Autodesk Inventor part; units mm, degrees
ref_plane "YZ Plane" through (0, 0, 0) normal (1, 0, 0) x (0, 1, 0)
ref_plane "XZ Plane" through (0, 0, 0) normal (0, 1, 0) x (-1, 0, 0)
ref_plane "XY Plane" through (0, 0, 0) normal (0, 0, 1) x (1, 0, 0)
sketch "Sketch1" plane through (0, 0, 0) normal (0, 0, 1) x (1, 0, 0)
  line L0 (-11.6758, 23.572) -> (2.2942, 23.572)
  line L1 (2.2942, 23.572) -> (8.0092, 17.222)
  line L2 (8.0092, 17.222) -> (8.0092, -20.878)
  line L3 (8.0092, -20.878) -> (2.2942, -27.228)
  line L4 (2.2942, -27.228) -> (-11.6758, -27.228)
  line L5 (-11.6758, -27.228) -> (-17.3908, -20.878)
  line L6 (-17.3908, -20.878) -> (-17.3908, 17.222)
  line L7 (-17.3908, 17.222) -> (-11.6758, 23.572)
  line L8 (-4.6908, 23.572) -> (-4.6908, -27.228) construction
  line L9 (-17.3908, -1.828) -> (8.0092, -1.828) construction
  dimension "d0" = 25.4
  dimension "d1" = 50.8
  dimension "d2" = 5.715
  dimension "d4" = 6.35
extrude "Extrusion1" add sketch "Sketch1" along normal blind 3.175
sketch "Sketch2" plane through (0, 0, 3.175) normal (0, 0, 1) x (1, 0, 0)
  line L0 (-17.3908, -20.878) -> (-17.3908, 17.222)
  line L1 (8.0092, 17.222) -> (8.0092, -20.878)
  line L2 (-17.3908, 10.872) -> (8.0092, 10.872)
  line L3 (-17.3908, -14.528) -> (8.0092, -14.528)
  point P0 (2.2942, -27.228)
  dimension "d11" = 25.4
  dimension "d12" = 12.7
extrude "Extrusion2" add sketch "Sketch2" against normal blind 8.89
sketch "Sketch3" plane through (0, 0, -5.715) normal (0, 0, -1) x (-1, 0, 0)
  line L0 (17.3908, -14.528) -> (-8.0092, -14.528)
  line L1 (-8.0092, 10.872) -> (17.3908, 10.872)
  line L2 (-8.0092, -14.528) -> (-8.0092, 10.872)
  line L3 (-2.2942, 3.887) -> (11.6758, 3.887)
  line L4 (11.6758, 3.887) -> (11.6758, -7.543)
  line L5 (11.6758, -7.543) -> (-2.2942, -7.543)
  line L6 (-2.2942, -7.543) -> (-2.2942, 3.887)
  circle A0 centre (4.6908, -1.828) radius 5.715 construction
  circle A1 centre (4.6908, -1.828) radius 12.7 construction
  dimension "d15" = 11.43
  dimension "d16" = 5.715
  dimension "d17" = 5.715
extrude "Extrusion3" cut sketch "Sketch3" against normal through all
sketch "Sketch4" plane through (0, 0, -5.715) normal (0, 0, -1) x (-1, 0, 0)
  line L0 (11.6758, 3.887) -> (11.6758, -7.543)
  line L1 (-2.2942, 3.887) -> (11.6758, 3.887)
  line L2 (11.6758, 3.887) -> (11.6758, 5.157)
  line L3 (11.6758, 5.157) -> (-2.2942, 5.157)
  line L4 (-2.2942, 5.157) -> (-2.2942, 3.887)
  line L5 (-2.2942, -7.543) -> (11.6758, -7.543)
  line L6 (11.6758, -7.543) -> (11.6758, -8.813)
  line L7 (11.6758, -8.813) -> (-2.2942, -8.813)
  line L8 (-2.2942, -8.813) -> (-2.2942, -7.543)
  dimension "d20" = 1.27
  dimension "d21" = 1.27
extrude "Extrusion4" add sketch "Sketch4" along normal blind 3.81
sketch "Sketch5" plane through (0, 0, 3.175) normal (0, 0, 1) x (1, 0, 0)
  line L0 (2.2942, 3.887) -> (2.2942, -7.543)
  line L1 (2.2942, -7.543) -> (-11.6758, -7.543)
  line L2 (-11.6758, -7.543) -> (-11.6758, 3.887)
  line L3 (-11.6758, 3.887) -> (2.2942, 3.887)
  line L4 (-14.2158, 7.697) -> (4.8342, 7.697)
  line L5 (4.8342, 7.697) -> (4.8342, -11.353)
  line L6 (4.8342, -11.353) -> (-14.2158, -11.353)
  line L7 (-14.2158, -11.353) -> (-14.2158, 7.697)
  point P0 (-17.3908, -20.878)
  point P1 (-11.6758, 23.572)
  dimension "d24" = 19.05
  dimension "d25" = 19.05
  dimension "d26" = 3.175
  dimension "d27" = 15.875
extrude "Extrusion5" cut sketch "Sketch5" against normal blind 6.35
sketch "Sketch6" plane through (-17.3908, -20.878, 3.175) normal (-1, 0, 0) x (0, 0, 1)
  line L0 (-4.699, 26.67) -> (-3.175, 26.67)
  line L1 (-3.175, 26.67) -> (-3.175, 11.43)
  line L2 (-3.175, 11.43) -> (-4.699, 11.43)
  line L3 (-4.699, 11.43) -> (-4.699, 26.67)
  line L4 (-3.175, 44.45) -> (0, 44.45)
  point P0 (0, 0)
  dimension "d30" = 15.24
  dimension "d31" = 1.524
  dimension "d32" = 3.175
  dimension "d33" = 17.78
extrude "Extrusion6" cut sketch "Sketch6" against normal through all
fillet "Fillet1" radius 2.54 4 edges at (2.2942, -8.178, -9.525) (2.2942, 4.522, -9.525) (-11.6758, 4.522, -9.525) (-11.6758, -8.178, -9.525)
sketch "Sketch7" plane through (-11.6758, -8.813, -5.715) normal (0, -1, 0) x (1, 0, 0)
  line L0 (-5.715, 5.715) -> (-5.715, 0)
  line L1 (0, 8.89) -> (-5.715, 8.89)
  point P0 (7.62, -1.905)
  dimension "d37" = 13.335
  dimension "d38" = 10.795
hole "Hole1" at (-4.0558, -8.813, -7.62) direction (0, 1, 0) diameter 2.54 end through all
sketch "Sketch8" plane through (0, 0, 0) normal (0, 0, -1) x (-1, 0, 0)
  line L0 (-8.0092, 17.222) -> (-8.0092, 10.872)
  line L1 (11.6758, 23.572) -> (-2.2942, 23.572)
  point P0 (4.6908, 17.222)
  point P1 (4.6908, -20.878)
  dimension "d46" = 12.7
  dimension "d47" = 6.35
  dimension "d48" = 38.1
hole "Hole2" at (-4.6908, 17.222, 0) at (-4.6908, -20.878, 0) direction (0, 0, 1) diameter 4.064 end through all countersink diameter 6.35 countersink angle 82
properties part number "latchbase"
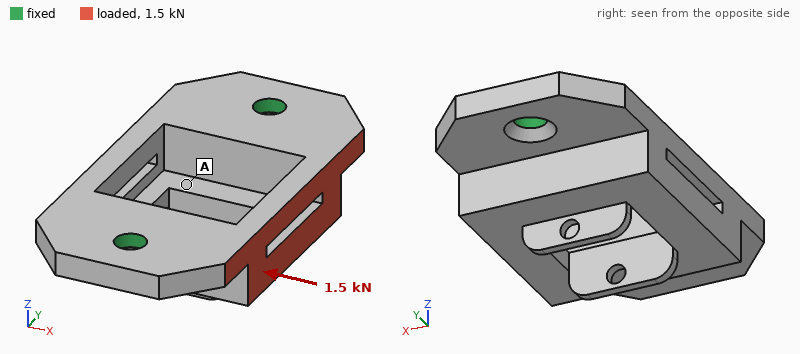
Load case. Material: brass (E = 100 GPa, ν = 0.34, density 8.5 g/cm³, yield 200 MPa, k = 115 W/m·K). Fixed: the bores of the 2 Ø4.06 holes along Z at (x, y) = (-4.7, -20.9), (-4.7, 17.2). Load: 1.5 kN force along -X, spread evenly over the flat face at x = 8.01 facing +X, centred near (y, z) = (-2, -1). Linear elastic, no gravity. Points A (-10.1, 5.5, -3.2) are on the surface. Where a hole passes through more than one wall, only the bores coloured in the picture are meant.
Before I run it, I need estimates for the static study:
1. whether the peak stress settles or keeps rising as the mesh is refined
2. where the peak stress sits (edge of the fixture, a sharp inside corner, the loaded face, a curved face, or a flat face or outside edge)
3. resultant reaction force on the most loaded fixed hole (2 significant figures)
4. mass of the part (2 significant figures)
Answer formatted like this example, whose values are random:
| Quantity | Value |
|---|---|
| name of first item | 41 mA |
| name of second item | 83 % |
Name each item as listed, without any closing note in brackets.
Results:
| Quantity | Value |
|---|---|
| whether the peak stress settles or keeps rising as the mesh is refined | keeps rising |
| where the peak stress sits | edge of the fixture |
| resultant reaction force on the most loaded fixed hole | 760 N |
| mass of the part | 40 g |
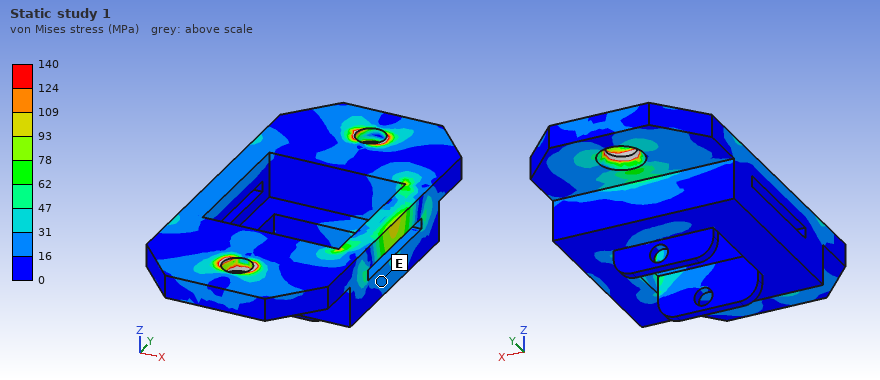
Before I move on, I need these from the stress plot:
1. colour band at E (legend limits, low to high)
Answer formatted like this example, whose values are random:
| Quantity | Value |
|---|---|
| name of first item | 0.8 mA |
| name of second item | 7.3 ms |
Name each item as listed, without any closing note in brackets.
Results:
| Quantity | Value |
|---|---|
| colour band at E | 16 to 31 MPa |
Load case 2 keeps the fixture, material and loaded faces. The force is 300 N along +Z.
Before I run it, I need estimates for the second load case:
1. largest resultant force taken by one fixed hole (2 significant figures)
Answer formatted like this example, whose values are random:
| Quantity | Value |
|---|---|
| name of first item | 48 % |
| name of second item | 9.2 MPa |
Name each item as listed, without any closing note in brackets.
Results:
| Quantity | Value |
|---|---|
| largest resultant force taken by one fixed hole | 210 N |
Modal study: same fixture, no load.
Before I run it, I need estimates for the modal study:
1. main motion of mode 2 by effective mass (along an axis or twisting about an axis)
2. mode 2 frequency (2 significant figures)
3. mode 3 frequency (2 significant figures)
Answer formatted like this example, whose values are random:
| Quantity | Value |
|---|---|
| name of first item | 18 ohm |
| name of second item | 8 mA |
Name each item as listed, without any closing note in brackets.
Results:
| Quantity | Value |
|---|---|
| main motion of mode 2 by effective mass | along Z |
| mode 2 frequency | 8500 Hz |
| mode 3 frequency | 9700 Hz |
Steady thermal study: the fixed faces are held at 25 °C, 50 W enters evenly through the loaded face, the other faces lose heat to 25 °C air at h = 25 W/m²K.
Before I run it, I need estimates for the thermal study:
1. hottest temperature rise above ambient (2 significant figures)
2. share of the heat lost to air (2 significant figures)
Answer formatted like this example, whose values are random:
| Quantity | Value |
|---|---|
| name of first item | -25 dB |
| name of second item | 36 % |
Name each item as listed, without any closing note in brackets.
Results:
| Quantity | Value |
|---|---|
| hottest temperature rise above ambient | 83 K |
| share of the heat lost to air | 5.3 % |
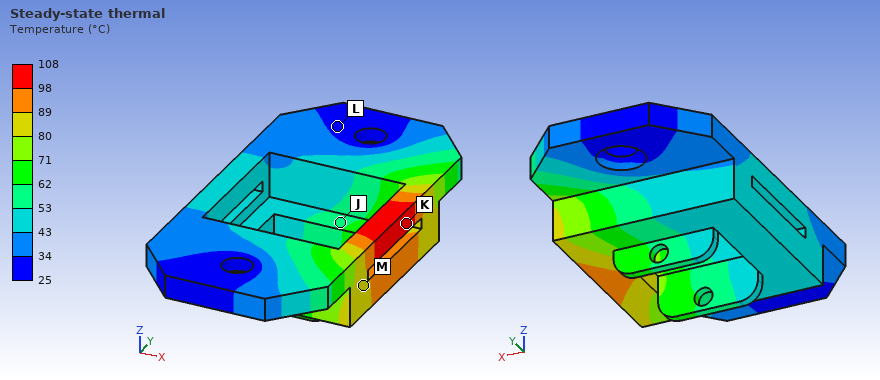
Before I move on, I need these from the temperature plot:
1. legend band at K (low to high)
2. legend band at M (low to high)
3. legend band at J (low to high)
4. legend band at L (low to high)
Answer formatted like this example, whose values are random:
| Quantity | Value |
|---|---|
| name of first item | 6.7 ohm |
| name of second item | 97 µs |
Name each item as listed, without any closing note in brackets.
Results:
| Quantity | Value |
|---|---|
| legend band at K | 98 to 108 °C |
| legend band at M | 80 to 89 °C |
| legend band at J | 53 to 62 °C |
| legend band at L | 25 to 34 °C |
